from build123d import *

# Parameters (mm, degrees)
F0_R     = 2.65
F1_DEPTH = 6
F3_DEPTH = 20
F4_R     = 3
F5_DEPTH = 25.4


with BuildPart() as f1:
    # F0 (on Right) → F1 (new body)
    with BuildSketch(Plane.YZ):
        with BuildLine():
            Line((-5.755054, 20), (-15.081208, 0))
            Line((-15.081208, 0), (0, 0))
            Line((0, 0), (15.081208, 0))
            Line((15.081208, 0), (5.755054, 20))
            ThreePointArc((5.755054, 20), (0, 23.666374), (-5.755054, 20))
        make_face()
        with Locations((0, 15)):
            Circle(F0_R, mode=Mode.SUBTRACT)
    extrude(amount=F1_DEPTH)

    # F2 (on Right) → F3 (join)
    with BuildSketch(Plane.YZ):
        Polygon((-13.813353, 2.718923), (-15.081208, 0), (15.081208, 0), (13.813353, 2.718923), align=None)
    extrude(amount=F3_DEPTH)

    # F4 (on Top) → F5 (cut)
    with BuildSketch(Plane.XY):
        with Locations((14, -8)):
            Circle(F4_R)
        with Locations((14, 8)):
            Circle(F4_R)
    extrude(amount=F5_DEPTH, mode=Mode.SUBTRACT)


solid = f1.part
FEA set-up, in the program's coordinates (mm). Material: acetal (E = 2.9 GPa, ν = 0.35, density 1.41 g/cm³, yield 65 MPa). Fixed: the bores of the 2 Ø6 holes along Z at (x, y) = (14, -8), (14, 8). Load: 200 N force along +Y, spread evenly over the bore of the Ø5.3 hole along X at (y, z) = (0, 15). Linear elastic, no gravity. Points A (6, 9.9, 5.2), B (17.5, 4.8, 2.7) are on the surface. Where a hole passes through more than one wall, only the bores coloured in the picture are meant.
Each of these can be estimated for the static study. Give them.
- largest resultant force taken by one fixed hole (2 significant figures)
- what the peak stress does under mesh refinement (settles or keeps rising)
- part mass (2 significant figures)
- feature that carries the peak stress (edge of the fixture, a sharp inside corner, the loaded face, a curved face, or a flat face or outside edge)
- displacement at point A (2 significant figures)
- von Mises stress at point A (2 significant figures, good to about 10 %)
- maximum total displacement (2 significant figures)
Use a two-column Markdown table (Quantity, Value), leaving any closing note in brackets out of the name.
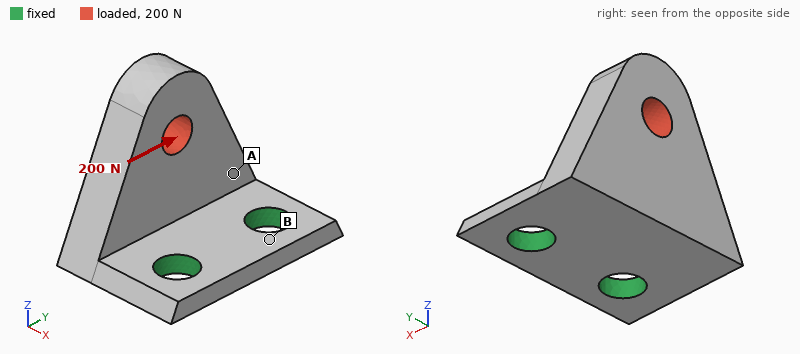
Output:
| Quantity | Value |
|---|---|
| largest resultant force taken by one fixed hole | 200 N |
| what the peak stress does under mesh refinement | keeps rising |
| part mass | 4.9 g |
| feature that carries the peak stress | edge of the fixture |
| displacement at point A | 0.16 mm |
| von Mises stress at point A | 13 MPa |
| maximum total displacement | 0.42 mm |
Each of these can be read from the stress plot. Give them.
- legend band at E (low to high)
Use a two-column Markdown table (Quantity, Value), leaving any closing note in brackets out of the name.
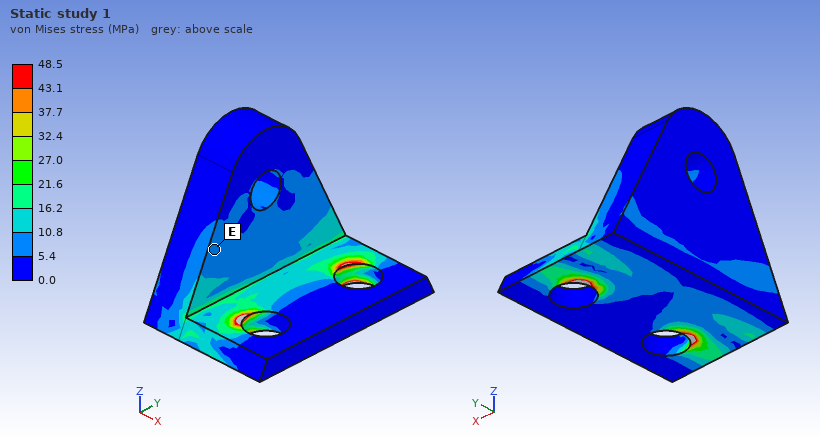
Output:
| Quantity | Value |
|---|---|
| legend band at E | 5.4 to 10.8 MPa |
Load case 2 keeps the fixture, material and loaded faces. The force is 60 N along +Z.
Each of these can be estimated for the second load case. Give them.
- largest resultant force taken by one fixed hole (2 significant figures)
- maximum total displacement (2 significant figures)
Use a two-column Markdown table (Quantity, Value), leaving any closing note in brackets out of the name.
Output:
| Quantity | Value |
|---|---|
| largest resultant force taken by one fixed hole | 30 N |
| maximum total displacement | 0.38 mm |
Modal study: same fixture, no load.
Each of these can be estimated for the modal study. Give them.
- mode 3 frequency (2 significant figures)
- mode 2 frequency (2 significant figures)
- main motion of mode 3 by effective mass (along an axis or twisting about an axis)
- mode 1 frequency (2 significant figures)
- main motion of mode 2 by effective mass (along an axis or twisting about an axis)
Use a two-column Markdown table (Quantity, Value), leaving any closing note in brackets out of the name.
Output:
| Quantity | Value |
|---|---|
| mode 3 frequency | 4400 Hz |
| mode 2 frequency | 2700 Hz |
| main motion of mode 3 by effective mass | along Z |
| mode 1 frequency | 1000 Hz |
| main motion of mode 2 by effective mass | along Y |
